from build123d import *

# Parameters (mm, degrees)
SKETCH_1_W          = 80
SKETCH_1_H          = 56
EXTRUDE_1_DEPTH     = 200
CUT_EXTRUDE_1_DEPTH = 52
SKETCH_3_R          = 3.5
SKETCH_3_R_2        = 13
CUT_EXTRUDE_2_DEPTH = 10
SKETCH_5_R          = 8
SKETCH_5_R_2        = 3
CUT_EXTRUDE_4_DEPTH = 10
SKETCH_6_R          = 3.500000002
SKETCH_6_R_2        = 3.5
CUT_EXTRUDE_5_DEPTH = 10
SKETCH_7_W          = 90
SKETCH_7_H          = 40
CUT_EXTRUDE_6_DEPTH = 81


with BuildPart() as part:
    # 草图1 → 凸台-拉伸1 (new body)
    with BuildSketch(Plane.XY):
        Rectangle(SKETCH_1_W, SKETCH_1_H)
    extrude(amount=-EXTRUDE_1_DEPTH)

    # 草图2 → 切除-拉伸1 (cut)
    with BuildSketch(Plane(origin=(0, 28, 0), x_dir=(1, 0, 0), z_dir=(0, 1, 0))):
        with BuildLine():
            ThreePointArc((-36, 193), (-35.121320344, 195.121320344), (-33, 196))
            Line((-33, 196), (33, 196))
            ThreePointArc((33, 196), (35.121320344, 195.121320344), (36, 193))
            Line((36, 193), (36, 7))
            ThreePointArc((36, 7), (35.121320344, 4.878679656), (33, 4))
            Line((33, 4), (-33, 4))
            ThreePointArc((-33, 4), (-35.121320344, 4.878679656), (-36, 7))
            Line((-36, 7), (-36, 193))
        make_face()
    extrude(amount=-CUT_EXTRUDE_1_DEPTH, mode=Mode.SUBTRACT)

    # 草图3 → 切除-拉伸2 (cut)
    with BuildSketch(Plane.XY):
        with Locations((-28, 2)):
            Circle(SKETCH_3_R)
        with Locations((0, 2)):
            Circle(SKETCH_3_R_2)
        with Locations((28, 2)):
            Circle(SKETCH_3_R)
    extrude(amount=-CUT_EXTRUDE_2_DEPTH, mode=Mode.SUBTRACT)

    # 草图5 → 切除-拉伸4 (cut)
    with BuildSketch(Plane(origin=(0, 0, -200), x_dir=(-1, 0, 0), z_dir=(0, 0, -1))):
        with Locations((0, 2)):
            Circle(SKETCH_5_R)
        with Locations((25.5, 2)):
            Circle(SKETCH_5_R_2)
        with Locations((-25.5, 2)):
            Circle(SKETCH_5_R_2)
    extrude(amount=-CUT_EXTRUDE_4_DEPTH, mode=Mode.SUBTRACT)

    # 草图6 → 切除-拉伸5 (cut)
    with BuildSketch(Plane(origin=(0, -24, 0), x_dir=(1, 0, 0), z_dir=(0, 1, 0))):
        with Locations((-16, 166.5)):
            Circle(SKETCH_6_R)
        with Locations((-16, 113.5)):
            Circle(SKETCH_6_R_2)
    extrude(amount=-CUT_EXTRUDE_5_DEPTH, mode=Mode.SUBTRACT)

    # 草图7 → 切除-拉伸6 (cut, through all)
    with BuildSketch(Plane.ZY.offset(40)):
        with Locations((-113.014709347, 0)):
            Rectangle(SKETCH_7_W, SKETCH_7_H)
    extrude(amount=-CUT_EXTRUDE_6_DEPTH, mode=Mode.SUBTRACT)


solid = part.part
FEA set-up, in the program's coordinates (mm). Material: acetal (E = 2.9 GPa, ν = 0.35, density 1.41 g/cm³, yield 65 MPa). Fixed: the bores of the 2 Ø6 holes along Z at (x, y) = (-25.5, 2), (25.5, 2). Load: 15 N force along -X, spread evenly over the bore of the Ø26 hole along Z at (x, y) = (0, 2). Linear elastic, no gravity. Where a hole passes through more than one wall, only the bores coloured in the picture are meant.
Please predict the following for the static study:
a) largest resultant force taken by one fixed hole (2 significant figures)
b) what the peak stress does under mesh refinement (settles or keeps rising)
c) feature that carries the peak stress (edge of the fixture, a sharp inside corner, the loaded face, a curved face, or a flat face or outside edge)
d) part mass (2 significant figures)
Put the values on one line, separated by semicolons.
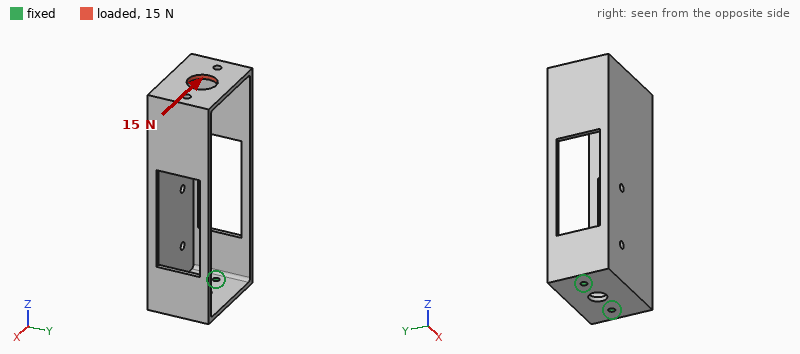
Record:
44 N; keeps rising; edge of the fixture; 200 g
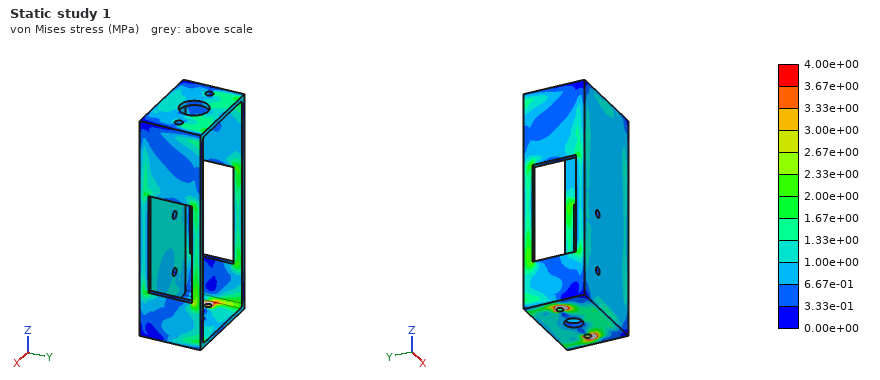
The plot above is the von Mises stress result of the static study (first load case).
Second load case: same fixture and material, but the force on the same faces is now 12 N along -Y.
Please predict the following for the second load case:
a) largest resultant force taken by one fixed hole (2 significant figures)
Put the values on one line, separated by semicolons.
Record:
6.3 N
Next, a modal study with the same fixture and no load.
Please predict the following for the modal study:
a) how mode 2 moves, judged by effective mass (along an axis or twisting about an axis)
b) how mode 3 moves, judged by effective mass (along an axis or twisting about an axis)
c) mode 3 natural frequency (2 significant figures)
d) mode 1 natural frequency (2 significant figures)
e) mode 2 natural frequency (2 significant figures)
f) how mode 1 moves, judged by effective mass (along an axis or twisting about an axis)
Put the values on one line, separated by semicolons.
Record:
along X; along X; 160 Hz; 41 Hz; 53 Hz; along Y
